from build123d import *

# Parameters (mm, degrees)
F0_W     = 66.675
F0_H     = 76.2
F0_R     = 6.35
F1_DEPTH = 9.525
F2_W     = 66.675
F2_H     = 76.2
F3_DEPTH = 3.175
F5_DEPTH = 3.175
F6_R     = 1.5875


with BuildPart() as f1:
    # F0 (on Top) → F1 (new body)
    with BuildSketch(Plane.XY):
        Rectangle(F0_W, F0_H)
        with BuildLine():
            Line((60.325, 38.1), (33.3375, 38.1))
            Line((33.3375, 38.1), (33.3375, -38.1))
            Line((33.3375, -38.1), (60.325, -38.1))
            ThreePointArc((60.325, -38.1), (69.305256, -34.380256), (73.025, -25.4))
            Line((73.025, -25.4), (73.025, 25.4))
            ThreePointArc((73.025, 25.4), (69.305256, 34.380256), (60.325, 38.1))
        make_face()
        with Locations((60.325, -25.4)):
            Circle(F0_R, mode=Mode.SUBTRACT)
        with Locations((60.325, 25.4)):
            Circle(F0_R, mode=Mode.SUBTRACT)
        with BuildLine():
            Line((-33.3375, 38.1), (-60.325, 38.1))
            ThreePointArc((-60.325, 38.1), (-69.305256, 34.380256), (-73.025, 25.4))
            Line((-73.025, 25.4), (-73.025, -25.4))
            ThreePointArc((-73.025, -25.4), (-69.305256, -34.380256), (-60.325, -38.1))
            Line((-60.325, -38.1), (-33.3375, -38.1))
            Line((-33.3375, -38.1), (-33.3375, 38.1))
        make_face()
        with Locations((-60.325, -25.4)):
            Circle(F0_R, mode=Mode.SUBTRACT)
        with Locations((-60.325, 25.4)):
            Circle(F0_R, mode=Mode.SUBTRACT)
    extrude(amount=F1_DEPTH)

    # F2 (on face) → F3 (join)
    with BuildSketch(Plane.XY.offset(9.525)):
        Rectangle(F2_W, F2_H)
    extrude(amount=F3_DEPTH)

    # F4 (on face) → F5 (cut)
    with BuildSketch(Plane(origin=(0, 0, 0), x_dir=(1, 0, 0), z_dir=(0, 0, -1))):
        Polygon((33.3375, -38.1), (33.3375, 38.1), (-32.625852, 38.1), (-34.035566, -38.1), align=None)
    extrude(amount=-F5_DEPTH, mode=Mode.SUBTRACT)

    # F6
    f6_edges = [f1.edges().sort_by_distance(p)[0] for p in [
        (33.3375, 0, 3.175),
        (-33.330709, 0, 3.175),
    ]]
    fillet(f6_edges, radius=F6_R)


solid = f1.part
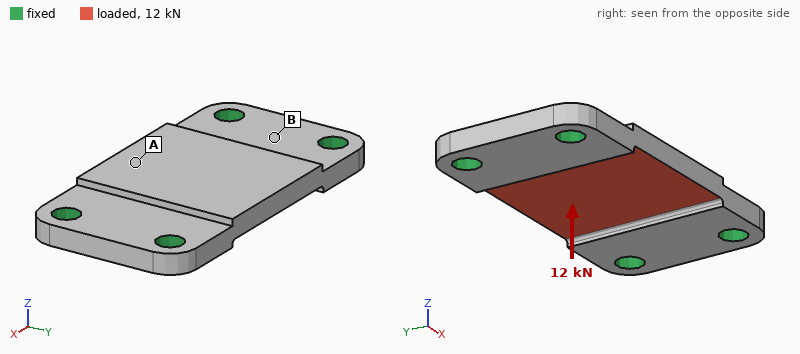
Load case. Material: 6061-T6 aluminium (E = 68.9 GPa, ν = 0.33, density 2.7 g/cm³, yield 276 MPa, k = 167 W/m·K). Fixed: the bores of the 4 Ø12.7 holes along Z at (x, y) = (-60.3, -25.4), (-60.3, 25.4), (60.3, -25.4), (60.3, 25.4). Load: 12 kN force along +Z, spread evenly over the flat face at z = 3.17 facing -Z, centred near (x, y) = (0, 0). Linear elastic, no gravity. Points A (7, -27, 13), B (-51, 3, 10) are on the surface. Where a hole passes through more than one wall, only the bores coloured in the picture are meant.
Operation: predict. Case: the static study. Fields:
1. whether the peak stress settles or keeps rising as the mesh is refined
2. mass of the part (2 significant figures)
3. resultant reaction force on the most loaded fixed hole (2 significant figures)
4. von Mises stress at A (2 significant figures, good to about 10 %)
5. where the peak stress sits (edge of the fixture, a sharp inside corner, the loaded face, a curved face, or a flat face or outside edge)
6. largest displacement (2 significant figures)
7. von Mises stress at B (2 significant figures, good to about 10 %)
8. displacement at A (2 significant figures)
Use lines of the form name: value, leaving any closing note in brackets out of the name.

whether the peak stress settles or keeps rising as the mesh is refined: keeps rising
mass of the part: 270 g
resultant reaction force on the most loaded fixed hole: 5.8 kN
von Mises stress at A: 79 MPa
where the peak stress sits: edge of the fixture
largest displacement: 0.19 mm
von Mises stress at B: 37 MPa
displacement at A: 0.17 mm
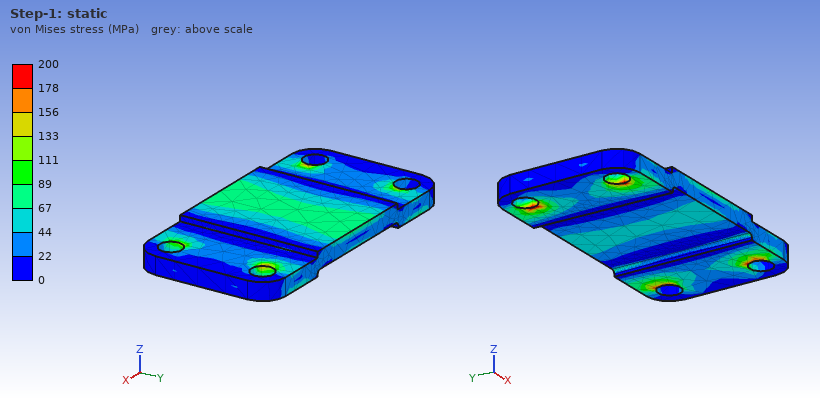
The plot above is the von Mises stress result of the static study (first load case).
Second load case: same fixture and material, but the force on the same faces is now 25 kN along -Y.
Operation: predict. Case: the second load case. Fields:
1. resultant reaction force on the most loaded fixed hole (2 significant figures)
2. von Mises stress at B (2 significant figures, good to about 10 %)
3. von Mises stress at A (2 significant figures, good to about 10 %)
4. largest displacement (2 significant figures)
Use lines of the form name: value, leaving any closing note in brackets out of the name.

resultant reaction force on the most loaded fixed hole: 7.8 kN
von Mises stress at B: 25 MPa
von Mises stress at A: 31 MPa
largest displacement: 74 µm
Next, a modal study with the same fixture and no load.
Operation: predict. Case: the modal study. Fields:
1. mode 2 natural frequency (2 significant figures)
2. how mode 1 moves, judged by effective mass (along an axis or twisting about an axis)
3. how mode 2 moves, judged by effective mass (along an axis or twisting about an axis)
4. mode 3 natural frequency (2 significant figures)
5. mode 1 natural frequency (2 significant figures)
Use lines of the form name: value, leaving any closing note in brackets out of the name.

mode 2 natural frequency: 5200 Hz
how mode 1 moves, judged by effective mass: along Z
how mode 2 moves, judged by effective mass: twisting about X
mode 3 natural frequency: 8900 Hz
mode 1 natural frequency: 3900 Hz
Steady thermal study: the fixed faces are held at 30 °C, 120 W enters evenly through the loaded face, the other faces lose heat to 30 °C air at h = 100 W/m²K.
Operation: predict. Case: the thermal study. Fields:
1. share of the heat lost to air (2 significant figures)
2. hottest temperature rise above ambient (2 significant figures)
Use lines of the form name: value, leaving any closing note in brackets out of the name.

share of the heat lost to air: 15 %
hottest temperature rise above ambient: 20 K
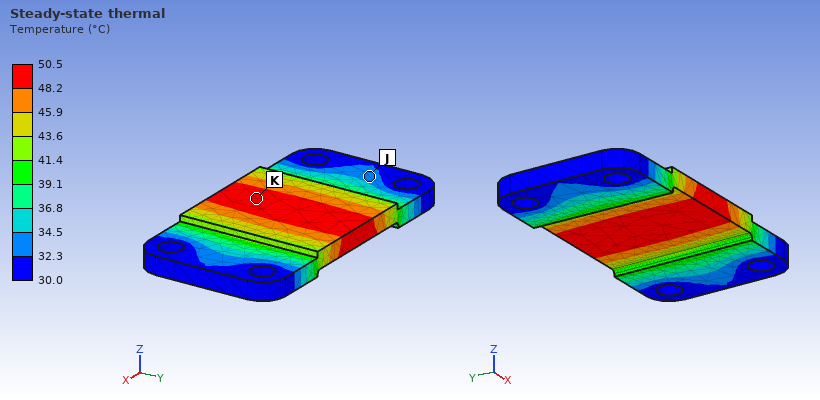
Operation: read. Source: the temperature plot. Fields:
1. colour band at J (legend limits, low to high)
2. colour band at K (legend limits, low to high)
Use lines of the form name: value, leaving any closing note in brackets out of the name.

colour band at J: 32.3 to 34.5 °C
colour band at K: 48.2 to 50.5 °C
